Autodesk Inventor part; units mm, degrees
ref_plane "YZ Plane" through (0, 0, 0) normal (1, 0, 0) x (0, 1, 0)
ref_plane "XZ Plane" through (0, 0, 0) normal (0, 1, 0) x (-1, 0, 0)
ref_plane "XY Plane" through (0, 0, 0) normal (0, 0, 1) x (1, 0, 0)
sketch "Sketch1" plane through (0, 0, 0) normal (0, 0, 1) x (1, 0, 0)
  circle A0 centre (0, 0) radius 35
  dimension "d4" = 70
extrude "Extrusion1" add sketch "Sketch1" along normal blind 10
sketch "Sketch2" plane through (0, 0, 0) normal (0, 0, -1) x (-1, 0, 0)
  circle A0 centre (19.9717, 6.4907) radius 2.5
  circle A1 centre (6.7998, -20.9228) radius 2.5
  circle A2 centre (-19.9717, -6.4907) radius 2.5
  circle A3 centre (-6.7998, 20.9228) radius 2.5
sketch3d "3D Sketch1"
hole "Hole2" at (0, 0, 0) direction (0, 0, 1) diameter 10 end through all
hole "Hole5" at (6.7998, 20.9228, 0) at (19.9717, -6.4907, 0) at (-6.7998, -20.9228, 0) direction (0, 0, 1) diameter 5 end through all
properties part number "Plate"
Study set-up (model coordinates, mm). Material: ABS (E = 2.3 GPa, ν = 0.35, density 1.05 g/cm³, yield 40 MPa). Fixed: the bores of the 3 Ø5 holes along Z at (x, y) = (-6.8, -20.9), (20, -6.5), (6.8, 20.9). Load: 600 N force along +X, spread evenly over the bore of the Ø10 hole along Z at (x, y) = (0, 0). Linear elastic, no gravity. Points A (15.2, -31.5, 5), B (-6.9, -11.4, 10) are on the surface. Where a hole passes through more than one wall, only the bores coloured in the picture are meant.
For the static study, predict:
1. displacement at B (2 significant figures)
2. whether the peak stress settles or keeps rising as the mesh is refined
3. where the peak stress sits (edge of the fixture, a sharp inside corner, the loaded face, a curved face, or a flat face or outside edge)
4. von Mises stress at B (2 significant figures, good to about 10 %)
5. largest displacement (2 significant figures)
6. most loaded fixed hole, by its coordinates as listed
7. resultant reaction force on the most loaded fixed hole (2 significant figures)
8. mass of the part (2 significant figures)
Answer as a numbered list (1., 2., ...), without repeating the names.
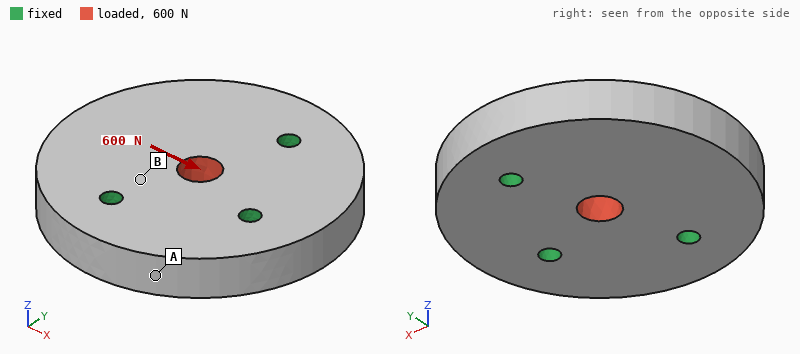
1. 7.0 µm
2. keeps rising
3. edge of the fixture
4. 0.79 MPa
5. 18 µm
6. (20, -6.5)
7. 240 N
8. 39 g
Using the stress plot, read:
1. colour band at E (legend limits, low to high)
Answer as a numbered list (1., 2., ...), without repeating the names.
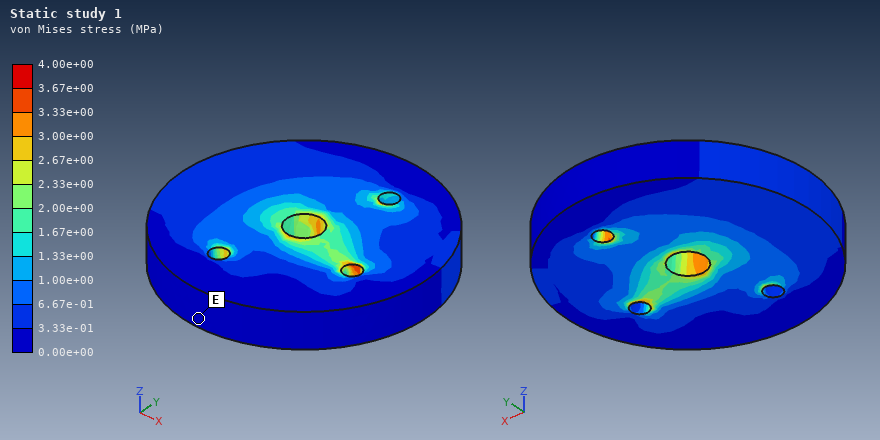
1. 0.00e+00 to 3.33e-01 MPa
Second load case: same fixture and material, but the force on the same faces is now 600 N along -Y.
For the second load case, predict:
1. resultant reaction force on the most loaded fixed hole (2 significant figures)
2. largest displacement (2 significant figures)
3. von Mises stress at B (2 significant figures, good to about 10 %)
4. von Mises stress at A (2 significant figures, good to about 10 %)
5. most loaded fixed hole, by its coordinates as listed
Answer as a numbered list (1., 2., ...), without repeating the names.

1. 270 N
2. 16 µm
3. 1.7 MPa
4. 0.36 MPa
5. (-6.8, -20.9)
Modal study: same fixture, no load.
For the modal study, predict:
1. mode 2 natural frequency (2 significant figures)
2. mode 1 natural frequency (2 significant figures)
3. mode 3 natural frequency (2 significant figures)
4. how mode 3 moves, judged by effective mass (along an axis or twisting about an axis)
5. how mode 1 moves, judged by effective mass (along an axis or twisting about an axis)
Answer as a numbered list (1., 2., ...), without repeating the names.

1. 4200 Hz
2. 2000 Hz
3. 5400 Hz
4. twisting about X
5. along Z
